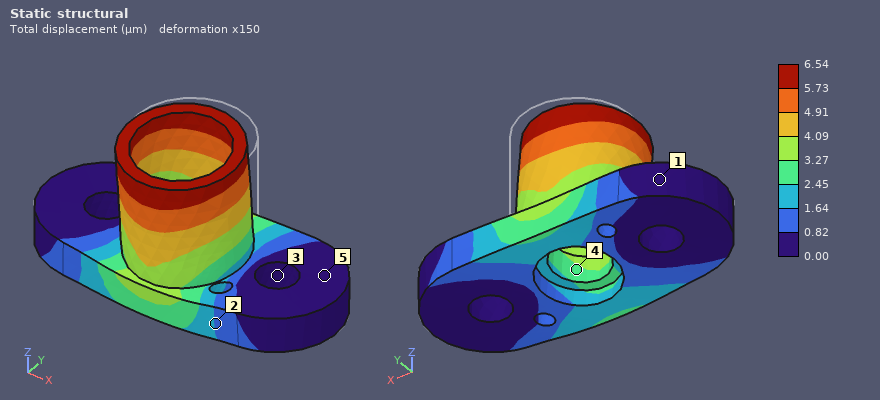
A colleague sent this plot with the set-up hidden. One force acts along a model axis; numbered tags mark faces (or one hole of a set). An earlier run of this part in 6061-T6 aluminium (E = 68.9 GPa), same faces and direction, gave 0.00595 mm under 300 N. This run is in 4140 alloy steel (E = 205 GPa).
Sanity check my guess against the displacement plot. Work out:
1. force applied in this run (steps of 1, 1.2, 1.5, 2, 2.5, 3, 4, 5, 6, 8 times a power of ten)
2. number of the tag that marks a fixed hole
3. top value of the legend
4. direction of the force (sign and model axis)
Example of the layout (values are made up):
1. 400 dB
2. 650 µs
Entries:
1. 1 kN
2. 3
3. 6.54 µm
4. -Y
